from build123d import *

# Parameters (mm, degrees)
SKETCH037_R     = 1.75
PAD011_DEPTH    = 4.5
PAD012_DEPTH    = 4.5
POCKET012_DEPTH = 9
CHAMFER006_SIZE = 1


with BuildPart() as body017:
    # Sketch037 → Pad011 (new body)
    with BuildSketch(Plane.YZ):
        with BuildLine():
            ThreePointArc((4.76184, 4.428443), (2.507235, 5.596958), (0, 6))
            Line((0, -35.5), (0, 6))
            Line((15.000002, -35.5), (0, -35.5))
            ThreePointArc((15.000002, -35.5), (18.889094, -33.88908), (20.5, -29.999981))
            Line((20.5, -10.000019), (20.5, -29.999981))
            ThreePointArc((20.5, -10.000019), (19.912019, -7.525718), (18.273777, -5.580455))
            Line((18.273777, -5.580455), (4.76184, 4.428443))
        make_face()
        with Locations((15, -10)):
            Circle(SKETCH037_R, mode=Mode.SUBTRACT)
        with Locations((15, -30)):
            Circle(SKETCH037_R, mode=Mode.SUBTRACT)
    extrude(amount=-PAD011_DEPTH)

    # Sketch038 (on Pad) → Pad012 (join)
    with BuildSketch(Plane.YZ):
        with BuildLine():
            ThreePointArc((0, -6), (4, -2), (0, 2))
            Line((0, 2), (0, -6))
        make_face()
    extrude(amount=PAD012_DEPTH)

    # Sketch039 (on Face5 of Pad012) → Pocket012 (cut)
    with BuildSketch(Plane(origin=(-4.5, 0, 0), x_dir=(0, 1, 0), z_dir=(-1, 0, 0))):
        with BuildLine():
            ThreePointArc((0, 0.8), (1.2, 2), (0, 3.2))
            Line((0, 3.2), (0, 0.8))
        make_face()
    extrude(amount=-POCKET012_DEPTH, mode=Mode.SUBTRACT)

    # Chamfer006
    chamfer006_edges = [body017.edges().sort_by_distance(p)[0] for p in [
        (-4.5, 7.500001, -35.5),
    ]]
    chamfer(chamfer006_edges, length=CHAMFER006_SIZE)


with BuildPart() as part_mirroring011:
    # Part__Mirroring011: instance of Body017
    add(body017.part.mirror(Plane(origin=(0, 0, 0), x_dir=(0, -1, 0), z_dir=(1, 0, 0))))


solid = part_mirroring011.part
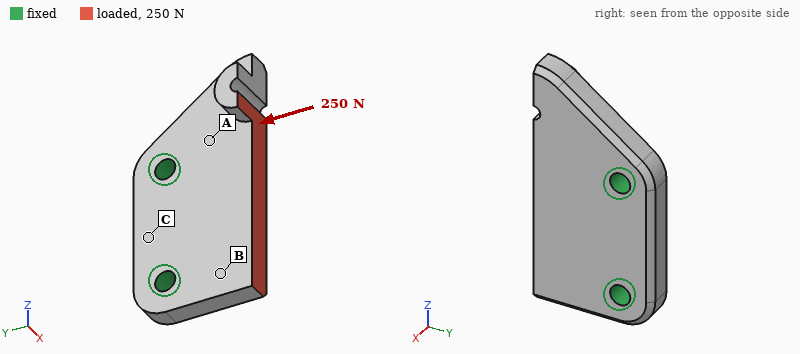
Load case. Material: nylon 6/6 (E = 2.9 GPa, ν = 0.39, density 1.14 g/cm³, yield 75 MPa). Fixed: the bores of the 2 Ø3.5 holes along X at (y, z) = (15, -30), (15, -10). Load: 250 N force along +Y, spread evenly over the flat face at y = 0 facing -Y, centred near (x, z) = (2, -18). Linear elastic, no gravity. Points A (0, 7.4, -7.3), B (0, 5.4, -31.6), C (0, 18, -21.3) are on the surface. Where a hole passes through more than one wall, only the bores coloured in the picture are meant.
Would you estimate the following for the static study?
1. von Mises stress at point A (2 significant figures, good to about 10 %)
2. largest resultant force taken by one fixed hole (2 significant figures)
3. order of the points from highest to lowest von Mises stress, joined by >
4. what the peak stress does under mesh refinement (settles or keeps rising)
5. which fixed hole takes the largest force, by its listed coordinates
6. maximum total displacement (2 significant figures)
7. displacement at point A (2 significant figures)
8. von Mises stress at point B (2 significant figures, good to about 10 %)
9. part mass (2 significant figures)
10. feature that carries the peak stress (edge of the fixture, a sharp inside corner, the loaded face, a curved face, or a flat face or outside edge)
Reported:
3.8 MPa
150 N
A > B > C
keeps rising
(15, -10)
68 µm
14 µm
1.8 MPa
3.7 g
edge of the fixture
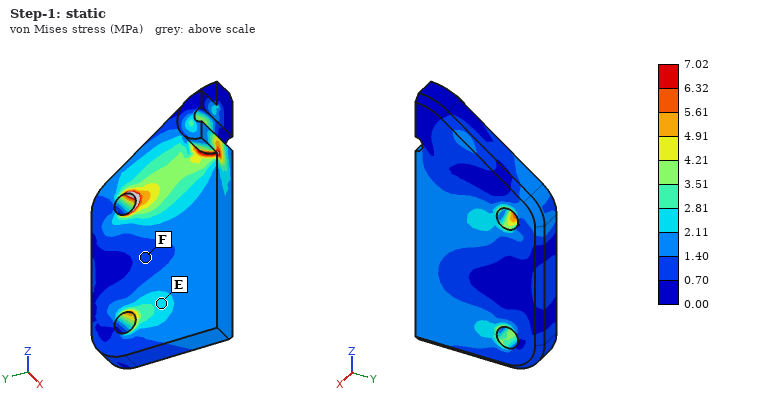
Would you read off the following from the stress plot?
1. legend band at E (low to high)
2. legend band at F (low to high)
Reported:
2.11 to 2.81 MPa
0.70 to 1.40 MPa
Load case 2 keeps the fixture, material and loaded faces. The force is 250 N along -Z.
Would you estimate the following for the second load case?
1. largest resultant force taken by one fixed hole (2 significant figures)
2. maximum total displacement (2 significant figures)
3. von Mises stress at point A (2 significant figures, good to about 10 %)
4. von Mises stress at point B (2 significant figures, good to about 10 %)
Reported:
210 N
91 µm
3.3 MPa
1.8 MPa
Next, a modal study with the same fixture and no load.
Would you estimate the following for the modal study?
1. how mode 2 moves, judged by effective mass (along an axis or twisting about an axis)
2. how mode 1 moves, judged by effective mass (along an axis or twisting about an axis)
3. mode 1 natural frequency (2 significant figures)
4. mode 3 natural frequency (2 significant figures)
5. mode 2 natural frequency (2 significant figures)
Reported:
along X
along X
3400 Hz
7800 Hz
4900 Hz
